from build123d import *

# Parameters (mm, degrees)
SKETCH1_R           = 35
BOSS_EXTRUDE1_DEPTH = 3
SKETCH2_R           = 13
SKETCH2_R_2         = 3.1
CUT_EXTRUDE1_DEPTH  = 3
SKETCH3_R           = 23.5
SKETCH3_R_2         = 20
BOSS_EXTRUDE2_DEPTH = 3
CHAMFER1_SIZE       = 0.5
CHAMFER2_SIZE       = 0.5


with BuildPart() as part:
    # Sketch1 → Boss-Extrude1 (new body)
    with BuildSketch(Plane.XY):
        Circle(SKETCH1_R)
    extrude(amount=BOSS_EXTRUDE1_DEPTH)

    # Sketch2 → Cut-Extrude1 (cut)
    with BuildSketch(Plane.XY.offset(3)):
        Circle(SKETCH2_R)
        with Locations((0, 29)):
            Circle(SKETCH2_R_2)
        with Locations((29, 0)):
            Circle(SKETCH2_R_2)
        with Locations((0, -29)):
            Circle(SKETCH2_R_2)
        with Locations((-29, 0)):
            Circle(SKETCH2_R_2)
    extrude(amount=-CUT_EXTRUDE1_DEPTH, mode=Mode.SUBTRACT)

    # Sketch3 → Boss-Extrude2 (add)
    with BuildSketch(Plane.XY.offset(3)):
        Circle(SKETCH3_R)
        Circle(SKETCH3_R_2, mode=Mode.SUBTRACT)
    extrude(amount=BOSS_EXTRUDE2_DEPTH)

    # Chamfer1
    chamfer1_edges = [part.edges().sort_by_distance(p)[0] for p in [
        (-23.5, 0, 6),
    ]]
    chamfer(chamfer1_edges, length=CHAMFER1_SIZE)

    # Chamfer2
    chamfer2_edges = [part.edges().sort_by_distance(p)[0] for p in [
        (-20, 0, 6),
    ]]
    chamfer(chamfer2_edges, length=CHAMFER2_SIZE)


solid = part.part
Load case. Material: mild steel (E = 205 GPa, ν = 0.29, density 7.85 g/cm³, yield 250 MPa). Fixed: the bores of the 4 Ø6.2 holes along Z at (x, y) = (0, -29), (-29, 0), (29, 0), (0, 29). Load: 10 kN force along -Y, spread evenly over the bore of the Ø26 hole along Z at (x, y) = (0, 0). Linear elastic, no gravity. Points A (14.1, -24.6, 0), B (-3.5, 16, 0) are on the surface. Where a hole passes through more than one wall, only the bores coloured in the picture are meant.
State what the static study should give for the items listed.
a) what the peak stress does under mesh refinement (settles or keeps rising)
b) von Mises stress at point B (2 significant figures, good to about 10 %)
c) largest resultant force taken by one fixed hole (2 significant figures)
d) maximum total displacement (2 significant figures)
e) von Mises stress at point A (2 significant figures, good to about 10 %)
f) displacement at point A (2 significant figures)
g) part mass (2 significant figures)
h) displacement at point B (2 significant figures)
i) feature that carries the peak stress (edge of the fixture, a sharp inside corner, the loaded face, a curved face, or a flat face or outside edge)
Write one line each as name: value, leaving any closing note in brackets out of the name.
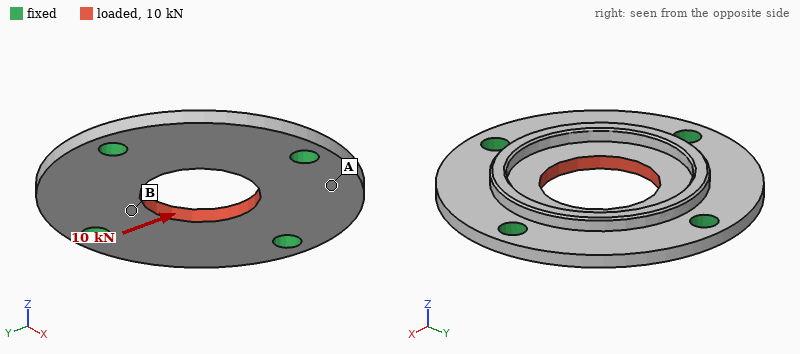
what the peak stress does under mesh refinement: keeps rising
von Mises stress at point B: 60 MPa
largest resultant force taken by one fixed hole: 2.9 kN
maximum total displacement: 6.2 µm
von Mises stress at point A: 16 MPa
displacement at point A: 3.4 µm
part mass: 86 g
displacement at point B: 3.6 µm
feature that carries the peak stress: edge of the fixture
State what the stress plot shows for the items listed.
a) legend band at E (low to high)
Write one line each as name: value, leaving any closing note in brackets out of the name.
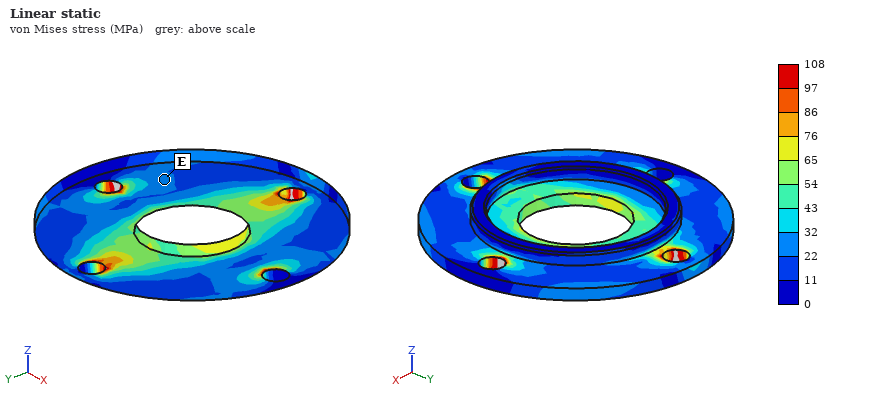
legend band at E: 22 to 32 MPa
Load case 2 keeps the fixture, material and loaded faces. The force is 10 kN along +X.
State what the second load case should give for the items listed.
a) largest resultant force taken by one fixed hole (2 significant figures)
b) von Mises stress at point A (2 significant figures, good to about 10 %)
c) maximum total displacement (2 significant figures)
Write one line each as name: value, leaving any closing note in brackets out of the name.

largest resultant force taken by one fixed hole: 2.9 kN
von Mises stress at point A: 22 MPa
maximum total displacement: 6.2 µm
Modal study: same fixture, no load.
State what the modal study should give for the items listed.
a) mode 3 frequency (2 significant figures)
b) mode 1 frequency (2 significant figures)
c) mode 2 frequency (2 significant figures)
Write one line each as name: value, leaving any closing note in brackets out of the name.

mode 3 frequency: 10000 Hz
mode 1 frequency: 9200 Hz
mode 2 frequency: 10000 Hz
